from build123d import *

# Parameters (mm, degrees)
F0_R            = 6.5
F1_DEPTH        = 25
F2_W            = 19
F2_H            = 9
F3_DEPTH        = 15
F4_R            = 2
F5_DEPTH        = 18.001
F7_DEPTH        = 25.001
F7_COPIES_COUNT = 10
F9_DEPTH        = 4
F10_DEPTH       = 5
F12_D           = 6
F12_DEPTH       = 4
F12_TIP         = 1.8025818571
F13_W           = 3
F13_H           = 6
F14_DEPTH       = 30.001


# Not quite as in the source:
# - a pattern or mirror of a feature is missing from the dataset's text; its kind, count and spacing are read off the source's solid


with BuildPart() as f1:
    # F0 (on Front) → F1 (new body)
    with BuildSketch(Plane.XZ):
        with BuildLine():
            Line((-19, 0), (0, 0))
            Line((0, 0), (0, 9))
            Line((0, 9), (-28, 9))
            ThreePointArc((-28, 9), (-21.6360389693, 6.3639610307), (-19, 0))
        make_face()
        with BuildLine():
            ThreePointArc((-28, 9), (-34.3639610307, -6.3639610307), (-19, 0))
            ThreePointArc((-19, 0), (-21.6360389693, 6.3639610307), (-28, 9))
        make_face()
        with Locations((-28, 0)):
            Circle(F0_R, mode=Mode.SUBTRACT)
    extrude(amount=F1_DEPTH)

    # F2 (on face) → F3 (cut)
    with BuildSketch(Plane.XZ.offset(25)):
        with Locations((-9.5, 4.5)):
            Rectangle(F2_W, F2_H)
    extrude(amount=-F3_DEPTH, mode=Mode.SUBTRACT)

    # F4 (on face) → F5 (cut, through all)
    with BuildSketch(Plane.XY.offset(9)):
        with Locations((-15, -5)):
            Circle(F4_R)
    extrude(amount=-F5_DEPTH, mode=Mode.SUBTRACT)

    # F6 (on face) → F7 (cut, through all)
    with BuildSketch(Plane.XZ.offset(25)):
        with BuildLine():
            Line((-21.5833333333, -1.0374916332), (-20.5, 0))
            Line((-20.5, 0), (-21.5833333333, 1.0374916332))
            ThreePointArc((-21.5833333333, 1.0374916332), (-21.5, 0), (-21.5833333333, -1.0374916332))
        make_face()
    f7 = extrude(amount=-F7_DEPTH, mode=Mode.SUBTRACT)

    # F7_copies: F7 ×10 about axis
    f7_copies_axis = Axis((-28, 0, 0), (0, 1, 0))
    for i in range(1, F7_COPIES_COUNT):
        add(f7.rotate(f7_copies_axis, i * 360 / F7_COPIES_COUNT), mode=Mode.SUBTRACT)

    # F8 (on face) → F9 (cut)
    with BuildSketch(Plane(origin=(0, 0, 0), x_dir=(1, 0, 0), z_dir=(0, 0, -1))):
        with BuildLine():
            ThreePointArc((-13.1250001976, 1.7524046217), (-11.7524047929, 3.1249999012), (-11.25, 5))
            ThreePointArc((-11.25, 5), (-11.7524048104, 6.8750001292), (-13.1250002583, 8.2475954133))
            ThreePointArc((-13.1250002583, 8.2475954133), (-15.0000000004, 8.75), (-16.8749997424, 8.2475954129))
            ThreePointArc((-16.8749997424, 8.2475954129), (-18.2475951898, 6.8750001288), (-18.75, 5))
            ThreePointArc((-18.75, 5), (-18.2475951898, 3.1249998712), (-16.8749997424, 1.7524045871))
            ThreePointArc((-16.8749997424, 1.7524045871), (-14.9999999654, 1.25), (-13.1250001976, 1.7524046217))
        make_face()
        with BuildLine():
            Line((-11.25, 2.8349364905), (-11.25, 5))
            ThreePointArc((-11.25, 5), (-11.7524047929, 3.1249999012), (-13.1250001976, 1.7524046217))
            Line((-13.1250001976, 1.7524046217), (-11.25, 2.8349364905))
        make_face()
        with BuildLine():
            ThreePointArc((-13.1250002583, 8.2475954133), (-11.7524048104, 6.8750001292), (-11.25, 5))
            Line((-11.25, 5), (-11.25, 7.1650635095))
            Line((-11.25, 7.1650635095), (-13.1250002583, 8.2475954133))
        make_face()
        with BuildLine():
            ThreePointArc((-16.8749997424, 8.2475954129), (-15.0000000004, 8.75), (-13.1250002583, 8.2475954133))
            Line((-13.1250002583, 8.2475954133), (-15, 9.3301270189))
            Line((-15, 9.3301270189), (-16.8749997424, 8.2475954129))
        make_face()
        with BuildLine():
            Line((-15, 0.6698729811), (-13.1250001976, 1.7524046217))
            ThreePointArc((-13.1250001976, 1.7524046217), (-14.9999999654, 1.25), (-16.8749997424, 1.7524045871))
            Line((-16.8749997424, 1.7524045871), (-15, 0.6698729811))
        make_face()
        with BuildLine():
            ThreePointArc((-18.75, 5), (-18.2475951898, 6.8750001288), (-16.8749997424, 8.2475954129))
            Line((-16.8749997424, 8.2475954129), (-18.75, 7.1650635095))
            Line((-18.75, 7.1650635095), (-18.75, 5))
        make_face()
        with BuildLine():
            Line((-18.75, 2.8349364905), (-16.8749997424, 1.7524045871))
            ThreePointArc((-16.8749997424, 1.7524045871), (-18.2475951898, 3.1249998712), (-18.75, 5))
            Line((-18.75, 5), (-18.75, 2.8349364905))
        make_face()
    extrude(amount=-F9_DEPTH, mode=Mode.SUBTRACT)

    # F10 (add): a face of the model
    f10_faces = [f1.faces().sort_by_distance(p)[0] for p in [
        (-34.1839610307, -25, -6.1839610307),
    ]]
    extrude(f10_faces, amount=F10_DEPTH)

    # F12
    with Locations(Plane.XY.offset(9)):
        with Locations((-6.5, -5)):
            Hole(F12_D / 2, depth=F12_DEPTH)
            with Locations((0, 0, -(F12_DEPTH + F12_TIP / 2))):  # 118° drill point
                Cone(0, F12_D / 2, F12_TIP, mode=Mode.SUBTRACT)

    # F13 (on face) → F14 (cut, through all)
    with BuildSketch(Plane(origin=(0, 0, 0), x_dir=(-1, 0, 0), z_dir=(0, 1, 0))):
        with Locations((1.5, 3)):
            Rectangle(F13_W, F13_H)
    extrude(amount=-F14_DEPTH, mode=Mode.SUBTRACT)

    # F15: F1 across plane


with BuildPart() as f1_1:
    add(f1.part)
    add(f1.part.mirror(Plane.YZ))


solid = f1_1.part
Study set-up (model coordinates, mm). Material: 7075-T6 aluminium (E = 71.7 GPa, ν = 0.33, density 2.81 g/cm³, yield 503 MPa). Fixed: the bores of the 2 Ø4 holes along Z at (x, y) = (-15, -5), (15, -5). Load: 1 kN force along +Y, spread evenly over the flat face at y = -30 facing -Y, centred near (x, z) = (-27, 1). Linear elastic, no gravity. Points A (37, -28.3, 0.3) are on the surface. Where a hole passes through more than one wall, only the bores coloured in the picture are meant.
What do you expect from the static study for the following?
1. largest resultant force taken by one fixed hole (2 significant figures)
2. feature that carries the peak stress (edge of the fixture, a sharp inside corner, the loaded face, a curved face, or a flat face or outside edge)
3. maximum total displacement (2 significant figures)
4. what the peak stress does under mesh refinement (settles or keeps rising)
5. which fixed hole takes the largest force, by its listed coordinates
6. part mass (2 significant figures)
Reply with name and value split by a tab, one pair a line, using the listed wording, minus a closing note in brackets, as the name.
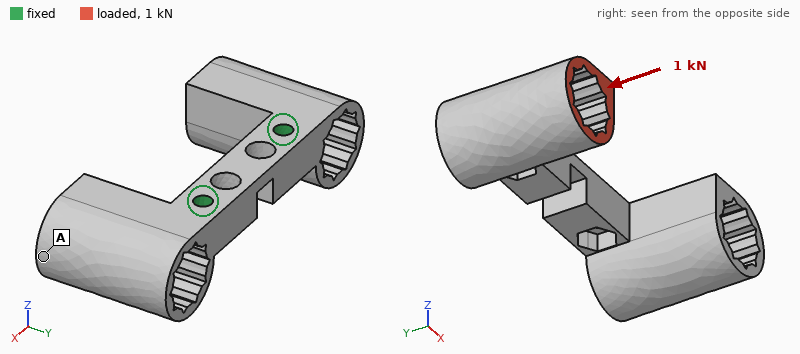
largest resultant force taken by one fixed hole	1.1 kN
feature that carries the peak stress	edge of the fixture
maximum total displacement	0.14 mm
what the peak stress does under mesh refinement	keeps rising
which fixed hole takes the largest force, by its listed coordinates	(-15, -5)
part mass	28 g
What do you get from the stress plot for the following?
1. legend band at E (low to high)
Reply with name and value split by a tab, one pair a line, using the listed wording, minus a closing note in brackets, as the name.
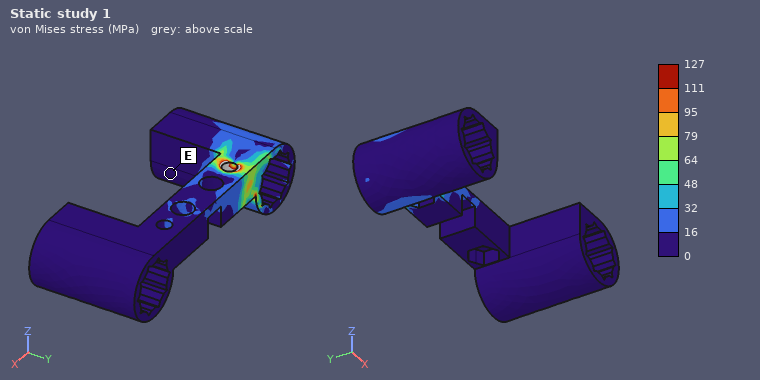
legend band at E	0 to 16 MPa
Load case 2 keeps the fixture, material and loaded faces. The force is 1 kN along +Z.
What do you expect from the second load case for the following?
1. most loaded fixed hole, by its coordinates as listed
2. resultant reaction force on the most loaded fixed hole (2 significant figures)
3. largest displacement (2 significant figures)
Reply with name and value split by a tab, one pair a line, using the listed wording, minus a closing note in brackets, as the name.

most loaded fixed hole, by its coordinates as listed	(-15, -5)
resultant reaction force on the most loaded fixed hole	1.1 kN
largest displacement	0.43 mm
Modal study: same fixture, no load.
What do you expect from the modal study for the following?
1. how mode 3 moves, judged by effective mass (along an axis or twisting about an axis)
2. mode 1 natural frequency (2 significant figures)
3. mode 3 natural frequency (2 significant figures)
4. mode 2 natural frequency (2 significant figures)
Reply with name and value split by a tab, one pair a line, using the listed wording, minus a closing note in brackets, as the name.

how mode 3 moves, judged by effective mass	along Y
mode 1 natural frequency	3600 Hz
mode 3 natural frequency	4200 Hz
mode 2 natural frequency	3600 Hz
